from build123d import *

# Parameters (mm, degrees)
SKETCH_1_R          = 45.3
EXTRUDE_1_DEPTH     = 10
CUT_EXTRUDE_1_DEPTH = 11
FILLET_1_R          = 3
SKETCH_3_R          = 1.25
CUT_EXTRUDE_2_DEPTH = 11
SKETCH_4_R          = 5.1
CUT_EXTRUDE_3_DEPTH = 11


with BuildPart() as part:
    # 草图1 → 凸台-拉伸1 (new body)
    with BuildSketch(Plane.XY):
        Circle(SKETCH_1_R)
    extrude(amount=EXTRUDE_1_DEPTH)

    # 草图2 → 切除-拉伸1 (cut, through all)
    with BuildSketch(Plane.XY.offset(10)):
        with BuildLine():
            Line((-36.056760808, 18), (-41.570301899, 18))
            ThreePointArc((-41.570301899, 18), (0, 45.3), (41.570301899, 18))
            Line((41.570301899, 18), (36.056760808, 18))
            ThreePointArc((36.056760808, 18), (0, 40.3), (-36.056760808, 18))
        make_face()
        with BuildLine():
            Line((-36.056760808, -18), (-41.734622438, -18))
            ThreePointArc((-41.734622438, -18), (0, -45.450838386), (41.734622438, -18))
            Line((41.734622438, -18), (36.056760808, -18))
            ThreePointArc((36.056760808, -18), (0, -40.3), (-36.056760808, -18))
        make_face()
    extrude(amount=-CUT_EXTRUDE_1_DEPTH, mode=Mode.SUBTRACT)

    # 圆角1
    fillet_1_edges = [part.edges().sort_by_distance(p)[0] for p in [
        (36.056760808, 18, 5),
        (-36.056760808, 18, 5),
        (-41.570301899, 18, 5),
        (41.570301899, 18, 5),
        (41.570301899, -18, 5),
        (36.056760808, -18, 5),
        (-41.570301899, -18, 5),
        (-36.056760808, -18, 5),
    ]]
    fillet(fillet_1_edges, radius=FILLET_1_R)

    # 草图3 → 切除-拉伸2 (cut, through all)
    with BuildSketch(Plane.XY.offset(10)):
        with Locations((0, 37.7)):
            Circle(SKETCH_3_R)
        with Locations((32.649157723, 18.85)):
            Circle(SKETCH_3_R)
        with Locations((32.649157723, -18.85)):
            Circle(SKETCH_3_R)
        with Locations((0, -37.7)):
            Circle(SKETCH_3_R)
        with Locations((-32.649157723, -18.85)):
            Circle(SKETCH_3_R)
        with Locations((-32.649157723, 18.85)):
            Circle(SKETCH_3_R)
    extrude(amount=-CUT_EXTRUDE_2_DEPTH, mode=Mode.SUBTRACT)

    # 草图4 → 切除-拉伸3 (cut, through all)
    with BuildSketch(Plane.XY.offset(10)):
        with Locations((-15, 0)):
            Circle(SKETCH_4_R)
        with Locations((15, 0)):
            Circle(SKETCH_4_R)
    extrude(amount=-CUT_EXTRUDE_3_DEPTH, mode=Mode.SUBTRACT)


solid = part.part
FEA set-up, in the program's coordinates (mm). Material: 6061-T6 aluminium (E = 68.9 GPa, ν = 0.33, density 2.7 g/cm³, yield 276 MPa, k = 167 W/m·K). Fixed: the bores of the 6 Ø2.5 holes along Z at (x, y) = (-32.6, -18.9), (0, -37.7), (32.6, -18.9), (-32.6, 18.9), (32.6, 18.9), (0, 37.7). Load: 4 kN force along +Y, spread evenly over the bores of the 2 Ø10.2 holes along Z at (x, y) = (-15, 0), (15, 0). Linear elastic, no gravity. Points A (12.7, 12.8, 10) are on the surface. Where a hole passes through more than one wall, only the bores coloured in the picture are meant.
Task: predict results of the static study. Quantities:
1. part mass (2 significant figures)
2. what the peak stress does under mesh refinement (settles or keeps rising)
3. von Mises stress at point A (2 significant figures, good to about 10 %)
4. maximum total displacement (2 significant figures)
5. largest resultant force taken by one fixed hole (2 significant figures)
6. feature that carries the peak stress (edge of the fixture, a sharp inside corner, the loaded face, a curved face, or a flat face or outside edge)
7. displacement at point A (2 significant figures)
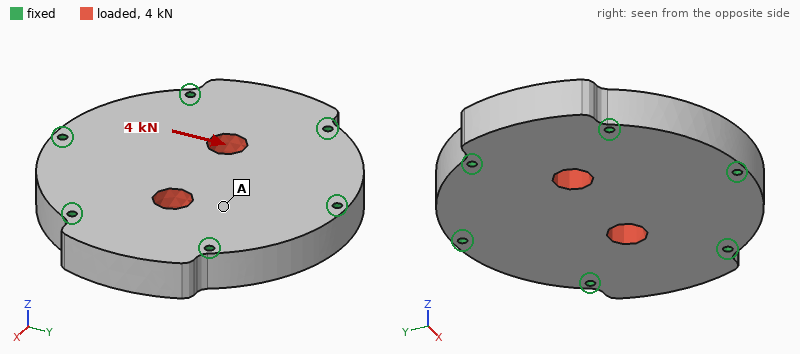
140 g
keeps rising
3.7 MPa
2.7 µm
790 N
edge of the fixture
2.0 µm
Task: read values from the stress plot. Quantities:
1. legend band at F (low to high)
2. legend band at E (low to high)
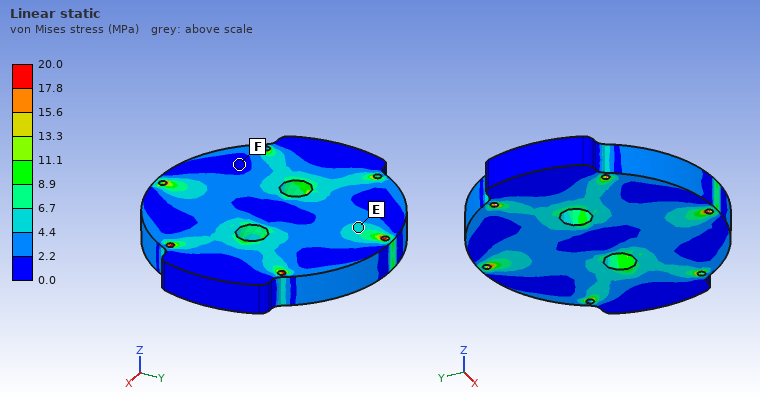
0.0 to 2.2 MPa
4.4 to 6.7 MPa
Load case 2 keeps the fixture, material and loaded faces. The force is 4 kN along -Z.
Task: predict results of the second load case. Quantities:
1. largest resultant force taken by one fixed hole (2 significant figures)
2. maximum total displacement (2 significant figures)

790 N
26 µm
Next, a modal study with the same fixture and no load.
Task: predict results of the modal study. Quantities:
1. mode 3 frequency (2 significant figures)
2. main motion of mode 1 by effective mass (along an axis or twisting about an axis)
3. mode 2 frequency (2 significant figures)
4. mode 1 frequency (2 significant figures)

20 kHz
along Z
19 kHz
11 kHz
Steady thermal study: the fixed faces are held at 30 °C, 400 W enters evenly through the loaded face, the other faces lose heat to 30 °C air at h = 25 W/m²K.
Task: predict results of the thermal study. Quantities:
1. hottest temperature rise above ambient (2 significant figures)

63 K
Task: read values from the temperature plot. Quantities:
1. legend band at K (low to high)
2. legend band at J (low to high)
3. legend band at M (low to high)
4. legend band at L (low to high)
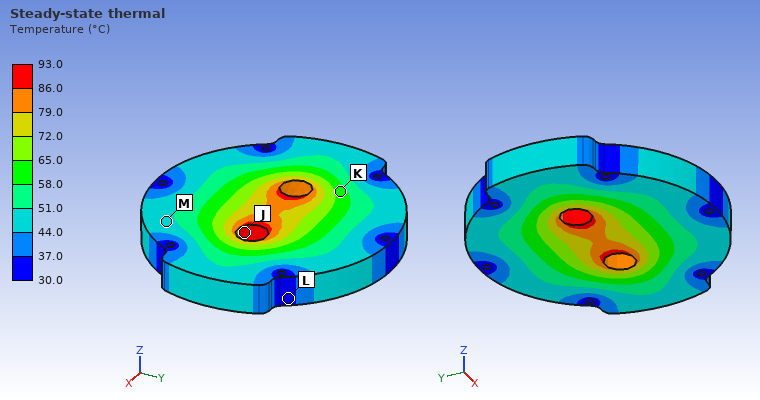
58.0 to 65.0 °C
86.0 to 93.0 °C
44.0 to 51.0 °C
30.0 to 37.0 °C
